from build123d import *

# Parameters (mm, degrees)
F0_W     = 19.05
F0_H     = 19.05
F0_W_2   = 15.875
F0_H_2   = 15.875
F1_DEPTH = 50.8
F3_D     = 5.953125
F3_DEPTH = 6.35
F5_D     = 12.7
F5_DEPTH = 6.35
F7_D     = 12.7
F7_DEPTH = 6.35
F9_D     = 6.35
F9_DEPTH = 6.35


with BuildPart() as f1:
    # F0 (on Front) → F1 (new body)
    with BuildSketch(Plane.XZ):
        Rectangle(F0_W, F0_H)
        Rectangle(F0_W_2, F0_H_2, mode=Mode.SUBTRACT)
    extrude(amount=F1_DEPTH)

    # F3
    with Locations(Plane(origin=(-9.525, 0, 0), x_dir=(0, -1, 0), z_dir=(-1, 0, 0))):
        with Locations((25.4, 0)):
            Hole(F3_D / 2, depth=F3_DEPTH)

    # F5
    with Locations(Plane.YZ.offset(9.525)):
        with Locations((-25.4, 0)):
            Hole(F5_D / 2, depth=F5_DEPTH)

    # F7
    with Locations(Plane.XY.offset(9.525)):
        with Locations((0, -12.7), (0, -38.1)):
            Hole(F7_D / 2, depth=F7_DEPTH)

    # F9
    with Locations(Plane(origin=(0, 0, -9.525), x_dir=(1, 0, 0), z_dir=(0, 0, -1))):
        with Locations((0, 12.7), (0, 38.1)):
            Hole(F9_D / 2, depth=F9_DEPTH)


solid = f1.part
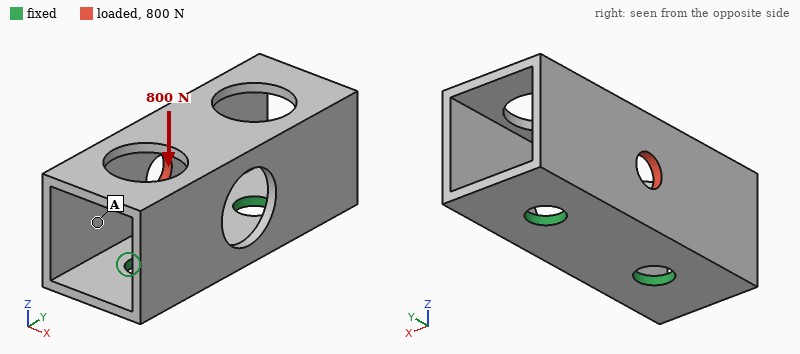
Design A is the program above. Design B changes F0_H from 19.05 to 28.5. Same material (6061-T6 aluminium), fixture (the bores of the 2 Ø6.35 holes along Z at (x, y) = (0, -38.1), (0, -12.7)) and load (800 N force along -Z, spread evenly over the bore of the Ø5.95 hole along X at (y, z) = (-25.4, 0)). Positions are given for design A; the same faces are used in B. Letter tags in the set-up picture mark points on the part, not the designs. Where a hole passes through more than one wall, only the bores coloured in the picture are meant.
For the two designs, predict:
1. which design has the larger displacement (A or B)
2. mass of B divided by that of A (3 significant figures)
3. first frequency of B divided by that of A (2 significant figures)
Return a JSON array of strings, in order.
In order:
["A", "2.57", "1.2"]
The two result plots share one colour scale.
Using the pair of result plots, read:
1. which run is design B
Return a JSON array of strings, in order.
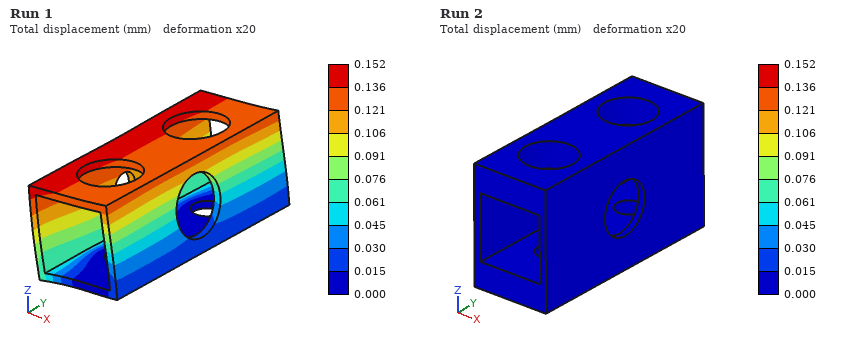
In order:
["Run 2"]
